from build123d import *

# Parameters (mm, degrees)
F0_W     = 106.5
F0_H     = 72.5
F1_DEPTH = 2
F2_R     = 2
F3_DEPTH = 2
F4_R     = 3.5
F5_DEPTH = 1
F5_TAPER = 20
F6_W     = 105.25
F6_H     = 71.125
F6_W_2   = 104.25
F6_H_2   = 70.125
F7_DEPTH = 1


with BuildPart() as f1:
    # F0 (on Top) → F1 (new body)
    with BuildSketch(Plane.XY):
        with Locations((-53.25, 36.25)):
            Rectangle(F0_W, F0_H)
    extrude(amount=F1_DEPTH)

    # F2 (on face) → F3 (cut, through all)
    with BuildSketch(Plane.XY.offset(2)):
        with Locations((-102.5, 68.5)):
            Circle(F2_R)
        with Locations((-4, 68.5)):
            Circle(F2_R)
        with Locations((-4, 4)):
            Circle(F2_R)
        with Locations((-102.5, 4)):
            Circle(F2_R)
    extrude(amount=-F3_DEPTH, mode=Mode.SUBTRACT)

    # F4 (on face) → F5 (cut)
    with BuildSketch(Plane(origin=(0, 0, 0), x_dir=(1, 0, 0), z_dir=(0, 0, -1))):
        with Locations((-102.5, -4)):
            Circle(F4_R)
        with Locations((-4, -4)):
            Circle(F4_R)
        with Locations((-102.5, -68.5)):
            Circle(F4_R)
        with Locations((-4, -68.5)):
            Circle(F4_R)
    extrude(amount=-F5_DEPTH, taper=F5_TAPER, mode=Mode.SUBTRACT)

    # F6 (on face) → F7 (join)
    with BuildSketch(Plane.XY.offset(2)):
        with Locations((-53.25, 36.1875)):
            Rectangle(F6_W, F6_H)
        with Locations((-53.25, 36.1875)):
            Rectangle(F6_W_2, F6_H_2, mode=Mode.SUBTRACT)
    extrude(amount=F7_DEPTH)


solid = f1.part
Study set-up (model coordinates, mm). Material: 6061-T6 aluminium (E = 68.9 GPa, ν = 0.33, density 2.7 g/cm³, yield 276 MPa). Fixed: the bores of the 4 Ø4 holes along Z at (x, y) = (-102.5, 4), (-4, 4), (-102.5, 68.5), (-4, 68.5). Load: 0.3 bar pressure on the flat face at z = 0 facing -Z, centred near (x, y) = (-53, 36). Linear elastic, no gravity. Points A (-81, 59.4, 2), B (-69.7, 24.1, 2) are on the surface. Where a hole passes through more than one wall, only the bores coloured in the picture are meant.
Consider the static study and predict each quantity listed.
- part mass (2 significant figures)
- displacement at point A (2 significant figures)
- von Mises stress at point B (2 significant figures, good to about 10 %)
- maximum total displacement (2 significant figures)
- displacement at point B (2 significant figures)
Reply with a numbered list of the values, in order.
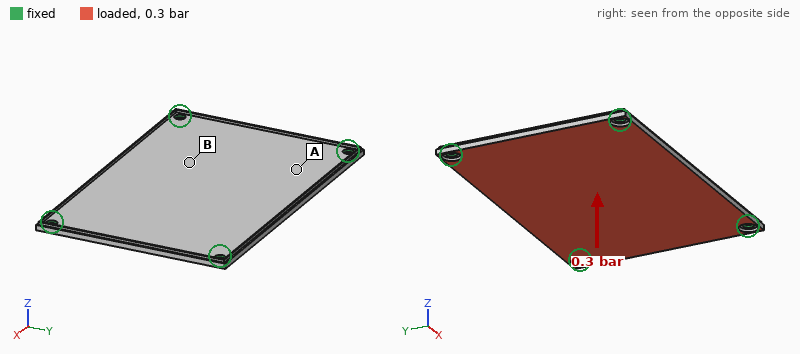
1. 42 g
2. 0.16 mm
3. 16 MPa
4. 0.30 mm
5. 0.25 mm
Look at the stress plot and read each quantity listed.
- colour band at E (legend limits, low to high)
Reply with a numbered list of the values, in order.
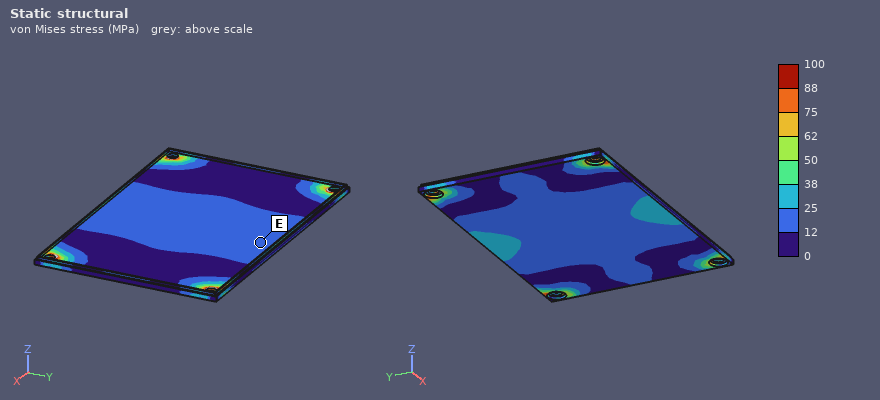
1. 12 to 25 MPa
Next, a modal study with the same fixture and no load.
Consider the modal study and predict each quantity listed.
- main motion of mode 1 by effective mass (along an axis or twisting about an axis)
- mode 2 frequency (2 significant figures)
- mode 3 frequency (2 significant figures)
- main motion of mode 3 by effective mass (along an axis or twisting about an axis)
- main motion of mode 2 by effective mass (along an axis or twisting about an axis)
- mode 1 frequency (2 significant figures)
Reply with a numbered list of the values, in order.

1. along Z
2. 1400 Hz
3. 2000 Hz
4. twisting about Y
5. twisting about X
6. 790 Hz
